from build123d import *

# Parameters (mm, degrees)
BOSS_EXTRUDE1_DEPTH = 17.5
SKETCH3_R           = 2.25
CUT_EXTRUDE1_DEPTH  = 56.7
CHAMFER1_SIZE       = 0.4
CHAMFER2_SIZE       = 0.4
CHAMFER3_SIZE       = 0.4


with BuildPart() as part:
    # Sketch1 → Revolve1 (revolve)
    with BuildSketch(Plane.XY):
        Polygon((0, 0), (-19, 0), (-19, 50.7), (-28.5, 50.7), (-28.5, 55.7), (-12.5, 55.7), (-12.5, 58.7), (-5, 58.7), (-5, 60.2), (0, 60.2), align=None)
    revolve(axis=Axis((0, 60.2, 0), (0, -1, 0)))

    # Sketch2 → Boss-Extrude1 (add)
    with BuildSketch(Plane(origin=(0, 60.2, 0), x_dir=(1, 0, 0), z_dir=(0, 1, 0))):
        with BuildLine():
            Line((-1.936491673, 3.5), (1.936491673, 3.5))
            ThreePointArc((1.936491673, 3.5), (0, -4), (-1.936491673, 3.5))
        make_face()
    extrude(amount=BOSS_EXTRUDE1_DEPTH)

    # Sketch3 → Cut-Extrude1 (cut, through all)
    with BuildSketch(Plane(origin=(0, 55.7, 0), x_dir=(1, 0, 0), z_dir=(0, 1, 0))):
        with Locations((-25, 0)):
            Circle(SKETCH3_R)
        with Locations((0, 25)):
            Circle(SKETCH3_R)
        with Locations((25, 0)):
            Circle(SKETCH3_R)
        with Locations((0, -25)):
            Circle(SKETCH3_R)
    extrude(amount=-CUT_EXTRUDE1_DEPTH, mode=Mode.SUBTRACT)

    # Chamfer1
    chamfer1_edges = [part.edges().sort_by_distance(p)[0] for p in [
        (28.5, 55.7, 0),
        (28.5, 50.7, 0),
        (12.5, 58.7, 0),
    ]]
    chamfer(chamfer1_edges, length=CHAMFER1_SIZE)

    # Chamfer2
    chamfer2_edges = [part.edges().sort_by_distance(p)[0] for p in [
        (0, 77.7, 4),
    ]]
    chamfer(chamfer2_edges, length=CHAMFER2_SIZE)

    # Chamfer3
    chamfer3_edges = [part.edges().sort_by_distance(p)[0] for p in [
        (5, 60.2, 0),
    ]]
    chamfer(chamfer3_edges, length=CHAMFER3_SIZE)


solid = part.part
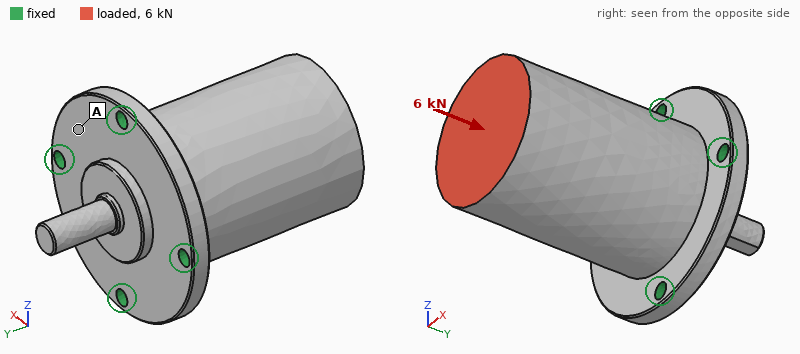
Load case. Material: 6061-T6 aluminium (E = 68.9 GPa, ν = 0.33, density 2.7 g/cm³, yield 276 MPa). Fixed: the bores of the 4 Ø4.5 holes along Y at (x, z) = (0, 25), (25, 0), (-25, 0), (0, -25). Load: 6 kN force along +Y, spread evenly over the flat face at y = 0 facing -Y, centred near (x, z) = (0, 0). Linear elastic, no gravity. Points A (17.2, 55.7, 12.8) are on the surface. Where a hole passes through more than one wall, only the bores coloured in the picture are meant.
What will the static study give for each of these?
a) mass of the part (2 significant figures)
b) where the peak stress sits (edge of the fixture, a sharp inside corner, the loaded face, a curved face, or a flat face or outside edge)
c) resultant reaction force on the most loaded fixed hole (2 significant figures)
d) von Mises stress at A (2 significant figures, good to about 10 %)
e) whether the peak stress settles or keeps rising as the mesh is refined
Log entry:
200 g
edge of the fixture
1.6 kN
16 MPa
keeps rising
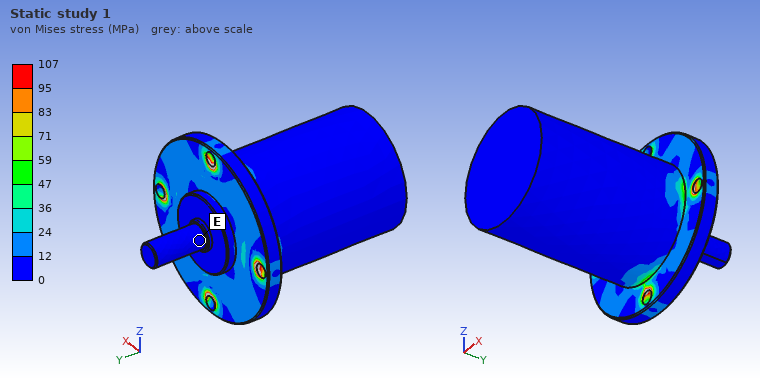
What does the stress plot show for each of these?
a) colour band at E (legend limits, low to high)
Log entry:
0 to 12 MPa
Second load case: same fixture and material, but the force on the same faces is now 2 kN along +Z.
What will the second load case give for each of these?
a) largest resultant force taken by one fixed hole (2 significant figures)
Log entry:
2.5 kN
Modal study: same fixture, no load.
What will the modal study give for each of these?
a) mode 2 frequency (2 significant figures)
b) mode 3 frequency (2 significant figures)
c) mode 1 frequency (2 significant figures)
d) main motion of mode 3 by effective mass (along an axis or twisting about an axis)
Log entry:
3800 Hz
7900 Hz
3800 Hz
along Y
